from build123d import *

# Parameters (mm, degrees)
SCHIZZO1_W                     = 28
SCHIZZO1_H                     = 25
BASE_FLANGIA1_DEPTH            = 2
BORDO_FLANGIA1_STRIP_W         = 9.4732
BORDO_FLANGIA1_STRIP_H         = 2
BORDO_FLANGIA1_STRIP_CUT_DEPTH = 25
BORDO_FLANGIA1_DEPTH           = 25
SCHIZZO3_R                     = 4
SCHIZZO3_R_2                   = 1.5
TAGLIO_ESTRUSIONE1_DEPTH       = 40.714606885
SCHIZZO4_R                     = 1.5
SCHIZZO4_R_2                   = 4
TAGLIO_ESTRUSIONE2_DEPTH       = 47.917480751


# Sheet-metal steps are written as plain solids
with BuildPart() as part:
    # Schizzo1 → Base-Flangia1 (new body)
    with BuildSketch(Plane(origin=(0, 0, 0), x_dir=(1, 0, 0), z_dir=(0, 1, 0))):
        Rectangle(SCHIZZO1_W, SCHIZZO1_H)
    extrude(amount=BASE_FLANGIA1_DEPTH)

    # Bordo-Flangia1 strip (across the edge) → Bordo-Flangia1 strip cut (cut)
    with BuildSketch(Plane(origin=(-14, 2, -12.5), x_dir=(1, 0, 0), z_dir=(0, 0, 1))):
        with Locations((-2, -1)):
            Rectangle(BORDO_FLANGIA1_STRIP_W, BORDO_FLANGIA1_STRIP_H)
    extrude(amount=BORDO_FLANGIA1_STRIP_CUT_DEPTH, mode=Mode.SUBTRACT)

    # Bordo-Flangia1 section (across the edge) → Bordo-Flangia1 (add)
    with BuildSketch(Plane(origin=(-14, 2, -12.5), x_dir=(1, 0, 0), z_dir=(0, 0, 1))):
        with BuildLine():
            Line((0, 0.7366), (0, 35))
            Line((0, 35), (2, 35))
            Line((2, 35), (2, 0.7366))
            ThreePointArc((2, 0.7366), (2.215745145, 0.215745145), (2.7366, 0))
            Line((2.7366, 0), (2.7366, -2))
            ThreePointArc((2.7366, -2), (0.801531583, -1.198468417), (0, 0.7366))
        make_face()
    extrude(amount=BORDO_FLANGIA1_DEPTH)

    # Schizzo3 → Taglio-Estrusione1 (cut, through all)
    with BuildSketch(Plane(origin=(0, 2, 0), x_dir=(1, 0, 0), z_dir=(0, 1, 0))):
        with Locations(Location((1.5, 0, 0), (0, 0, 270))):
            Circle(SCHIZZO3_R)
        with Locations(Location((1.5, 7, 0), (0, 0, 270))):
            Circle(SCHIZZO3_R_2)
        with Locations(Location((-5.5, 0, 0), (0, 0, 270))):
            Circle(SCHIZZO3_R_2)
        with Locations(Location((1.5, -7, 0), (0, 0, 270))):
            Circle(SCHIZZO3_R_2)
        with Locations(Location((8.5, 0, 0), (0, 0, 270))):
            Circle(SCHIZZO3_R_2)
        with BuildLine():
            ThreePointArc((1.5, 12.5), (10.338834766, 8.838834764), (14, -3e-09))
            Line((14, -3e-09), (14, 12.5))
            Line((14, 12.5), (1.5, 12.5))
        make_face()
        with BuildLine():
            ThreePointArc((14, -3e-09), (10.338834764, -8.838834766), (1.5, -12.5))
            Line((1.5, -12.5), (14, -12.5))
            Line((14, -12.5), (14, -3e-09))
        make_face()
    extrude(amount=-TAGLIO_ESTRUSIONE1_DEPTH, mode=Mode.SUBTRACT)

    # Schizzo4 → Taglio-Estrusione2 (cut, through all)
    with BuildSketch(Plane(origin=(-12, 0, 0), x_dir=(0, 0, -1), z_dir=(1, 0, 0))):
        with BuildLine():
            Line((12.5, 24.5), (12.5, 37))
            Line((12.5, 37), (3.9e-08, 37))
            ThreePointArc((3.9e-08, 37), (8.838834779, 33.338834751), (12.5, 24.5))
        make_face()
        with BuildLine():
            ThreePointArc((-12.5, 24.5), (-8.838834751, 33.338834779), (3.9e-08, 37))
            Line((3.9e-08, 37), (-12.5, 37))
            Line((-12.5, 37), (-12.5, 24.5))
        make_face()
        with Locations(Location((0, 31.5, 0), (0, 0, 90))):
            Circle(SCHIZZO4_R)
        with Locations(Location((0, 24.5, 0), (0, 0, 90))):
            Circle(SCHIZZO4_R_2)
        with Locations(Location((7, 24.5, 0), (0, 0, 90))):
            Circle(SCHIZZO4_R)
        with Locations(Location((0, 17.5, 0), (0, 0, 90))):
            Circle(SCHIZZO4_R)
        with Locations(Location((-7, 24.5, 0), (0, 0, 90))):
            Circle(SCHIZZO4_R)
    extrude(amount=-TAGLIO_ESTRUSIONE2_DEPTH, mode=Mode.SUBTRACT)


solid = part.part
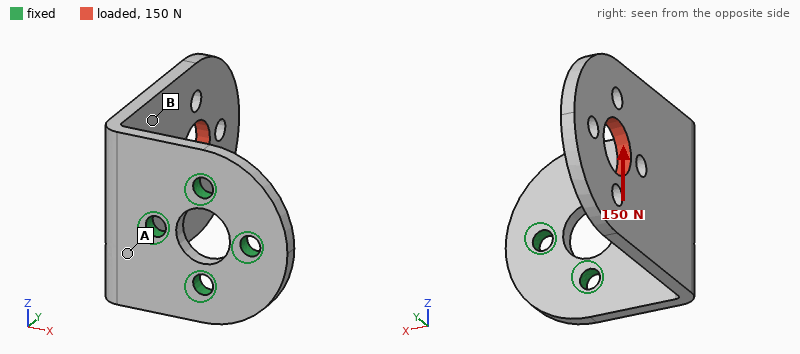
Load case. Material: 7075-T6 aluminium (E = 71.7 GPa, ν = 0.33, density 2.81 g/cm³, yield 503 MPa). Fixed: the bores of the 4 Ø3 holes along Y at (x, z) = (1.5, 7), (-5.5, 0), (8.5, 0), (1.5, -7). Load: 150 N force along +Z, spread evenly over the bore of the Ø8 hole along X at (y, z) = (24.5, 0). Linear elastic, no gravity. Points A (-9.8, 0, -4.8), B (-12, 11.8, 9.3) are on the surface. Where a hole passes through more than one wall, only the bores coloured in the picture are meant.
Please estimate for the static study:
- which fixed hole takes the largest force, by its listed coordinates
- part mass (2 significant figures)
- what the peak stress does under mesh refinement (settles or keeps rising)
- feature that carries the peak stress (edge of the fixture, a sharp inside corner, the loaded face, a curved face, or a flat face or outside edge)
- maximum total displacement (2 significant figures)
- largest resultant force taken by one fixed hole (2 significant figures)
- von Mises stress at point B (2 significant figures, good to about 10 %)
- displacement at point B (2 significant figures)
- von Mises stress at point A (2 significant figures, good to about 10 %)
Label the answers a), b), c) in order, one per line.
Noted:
a) (-5.5, 0)
b) 7.1 g
c) keeps rising
d) edge of the fixture
e) 0.39 mm
f) 140 N
g) 28 MPa
h) 0.16 mm
i) 71 MPa
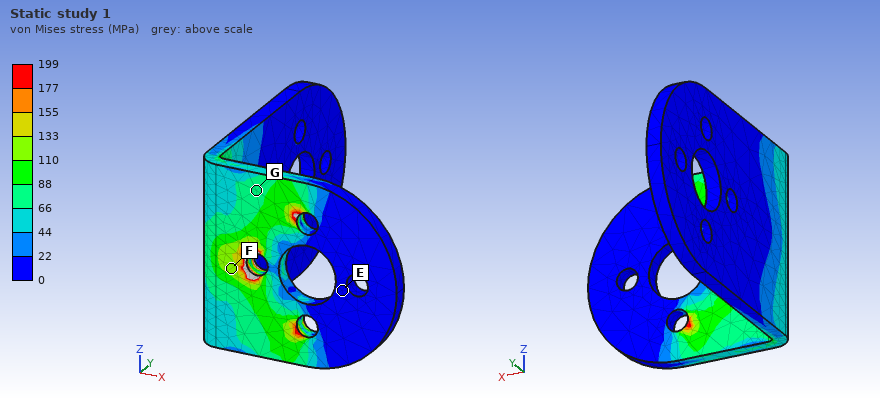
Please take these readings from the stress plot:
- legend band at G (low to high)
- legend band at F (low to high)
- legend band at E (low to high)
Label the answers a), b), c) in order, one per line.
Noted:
a) 66 to 88 MPa
b) 110 to 133 MPa
c) 0 to 22 MPa
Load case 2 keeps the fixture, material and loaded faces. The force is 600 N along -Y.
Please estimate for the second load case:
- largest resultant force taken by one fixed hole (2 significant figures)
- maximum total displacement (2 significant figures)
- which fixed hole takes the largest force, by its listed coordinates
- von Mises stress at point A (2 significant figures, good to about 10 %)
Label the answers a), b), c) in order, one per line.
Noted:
a) 740 N
b) 0.56 mm
c) (-5.5, 0)
d) 120 MPa
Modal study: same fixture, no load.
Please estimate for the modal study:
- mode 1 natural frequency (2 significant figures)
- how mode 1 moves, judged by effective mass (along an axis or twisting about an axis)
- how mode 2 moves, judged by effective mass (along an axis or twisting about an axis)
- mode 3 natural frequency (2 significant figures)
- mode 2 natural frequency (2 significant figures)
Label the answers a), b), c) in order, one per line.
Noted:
a) 1200 Hz
b) along X
c) along Z
d) 4500 Hz
e) 2200 Hz
